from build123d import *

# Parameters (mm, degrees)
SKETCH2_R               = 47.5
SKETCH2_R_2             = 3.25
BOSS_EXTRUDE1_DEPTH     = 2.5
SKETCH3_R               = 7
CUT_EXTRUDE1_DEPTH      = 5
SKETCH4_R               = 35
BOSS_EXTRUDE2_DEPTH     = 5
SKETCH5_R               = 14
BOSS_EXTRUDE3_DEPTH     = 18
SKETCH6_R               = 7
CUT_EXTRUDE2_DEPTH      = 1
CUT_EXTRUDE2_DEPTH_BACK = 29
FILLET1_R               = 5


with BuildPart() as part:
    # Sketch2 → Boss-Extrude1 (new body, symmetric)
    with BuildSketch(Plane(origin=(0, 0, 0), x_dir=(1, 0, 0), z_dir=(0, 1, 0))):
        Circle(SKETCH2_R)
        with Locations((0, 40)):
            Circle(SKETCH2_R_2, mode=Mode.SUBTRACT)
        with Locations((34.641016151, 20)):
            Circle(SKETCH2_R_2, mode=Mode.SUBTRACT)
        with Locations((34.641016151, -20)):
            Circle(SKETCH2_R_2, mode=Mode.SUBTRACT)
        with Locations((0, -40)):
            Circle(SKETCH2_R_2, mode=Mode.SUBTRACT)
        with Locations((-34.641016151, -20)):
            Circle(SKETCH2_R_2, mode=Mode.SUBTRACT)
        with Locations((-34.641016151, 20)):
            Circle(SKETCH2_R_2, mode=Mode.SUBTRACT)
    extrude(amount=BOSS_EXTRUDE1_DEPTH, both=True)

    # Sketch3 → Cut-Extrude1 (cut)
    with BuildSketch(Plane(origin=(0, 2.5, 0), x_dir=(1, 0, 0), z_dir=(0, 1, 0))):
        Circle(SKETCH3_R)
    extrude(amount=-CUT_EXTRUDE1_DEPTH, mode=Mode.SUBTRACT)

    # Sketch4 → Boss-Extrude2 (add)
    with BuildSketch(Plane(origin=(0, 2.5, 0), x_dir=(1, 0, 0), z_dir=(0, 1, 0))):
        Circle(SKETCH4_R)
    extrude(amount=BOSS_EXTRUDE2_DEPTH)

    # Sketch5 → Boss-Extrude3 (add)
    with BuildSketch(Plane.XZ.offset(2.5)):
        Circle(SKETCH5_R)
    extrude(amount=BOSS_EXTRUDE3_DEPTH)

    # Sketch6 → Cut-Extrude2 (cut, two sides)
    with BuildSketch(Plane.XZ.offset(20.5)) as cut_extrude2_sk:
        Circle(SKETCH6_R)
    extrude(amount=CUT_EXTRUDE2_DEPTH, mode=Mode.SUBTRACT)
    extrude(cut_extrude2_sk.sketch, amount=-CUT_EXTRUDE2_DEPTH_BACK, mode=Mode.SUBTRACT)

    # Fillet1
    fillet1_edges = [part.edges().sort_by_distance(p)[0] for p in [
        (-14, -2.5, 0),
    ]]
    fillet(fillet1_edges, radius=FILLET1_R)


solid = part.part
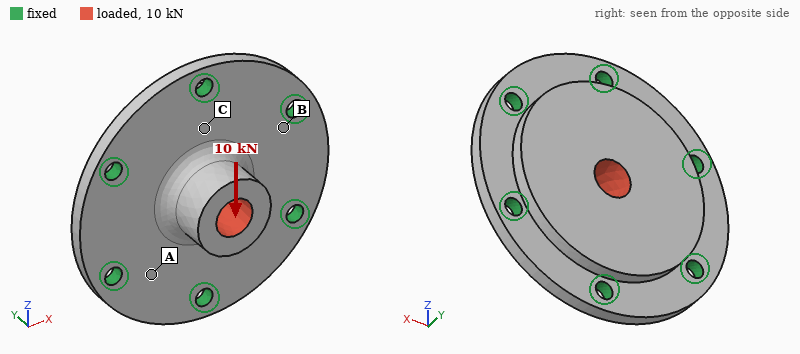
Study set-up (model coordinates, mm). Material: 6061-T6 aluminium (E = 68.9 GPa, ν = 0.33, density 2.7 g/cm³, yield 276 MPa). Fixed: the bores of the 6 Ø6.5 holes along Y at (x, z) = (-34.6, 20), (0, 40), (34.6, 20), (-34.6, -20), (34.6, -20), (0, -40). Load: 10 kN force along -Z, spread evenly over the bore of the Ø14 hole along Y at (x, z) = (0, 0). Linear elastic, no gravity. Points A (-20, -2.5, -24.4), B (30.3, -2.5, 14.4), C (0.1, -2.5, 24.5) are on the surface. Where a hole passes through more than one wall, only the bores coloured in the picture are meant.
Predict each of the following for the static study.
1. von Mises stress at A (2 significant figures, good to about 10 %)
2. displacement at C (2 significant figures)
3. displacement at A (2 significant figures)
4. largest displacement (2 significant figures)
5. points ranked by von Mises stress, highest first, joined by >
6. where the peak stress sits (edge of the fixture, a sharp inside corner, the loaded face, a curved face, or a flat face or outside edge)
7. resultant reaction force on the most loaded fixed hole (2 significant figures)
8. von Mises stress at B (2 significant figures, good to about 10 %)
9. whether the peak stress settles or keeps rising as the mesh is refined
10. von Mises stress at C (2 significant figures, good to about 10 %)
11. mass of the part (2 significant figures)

9.0 MPa
10.0 µm
6.6 µm
36 µm
C > B > A
edge of the fixture
2.3 kN
22 MPa
keeps rising
33 MPa
160 g
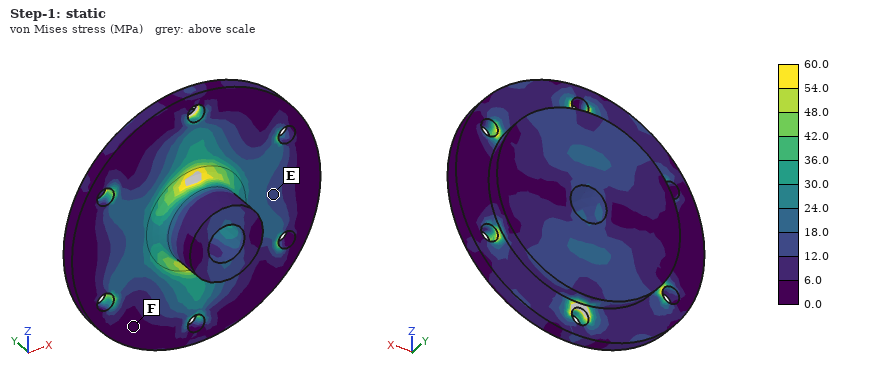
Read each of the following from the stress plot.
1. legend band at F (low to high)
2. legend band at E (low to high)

0.0 to 6.0 MPa
12.0 to 18.0 MPa
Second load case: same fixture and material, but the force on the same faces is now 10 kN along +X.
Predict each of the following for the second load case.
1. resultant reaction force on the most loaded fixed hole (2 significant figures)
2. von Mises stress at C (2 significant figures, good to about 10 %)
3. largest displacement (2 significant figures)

2.1 kN
14 MPa
36 µm
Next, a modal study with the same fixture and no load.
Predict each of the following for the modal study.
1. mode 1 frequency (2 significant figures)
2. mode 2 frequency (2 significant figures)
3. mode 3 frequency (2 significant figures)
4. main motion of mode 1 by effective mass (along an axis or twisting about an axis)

8600 Hz
13 kHz
13 kHz
along Y
